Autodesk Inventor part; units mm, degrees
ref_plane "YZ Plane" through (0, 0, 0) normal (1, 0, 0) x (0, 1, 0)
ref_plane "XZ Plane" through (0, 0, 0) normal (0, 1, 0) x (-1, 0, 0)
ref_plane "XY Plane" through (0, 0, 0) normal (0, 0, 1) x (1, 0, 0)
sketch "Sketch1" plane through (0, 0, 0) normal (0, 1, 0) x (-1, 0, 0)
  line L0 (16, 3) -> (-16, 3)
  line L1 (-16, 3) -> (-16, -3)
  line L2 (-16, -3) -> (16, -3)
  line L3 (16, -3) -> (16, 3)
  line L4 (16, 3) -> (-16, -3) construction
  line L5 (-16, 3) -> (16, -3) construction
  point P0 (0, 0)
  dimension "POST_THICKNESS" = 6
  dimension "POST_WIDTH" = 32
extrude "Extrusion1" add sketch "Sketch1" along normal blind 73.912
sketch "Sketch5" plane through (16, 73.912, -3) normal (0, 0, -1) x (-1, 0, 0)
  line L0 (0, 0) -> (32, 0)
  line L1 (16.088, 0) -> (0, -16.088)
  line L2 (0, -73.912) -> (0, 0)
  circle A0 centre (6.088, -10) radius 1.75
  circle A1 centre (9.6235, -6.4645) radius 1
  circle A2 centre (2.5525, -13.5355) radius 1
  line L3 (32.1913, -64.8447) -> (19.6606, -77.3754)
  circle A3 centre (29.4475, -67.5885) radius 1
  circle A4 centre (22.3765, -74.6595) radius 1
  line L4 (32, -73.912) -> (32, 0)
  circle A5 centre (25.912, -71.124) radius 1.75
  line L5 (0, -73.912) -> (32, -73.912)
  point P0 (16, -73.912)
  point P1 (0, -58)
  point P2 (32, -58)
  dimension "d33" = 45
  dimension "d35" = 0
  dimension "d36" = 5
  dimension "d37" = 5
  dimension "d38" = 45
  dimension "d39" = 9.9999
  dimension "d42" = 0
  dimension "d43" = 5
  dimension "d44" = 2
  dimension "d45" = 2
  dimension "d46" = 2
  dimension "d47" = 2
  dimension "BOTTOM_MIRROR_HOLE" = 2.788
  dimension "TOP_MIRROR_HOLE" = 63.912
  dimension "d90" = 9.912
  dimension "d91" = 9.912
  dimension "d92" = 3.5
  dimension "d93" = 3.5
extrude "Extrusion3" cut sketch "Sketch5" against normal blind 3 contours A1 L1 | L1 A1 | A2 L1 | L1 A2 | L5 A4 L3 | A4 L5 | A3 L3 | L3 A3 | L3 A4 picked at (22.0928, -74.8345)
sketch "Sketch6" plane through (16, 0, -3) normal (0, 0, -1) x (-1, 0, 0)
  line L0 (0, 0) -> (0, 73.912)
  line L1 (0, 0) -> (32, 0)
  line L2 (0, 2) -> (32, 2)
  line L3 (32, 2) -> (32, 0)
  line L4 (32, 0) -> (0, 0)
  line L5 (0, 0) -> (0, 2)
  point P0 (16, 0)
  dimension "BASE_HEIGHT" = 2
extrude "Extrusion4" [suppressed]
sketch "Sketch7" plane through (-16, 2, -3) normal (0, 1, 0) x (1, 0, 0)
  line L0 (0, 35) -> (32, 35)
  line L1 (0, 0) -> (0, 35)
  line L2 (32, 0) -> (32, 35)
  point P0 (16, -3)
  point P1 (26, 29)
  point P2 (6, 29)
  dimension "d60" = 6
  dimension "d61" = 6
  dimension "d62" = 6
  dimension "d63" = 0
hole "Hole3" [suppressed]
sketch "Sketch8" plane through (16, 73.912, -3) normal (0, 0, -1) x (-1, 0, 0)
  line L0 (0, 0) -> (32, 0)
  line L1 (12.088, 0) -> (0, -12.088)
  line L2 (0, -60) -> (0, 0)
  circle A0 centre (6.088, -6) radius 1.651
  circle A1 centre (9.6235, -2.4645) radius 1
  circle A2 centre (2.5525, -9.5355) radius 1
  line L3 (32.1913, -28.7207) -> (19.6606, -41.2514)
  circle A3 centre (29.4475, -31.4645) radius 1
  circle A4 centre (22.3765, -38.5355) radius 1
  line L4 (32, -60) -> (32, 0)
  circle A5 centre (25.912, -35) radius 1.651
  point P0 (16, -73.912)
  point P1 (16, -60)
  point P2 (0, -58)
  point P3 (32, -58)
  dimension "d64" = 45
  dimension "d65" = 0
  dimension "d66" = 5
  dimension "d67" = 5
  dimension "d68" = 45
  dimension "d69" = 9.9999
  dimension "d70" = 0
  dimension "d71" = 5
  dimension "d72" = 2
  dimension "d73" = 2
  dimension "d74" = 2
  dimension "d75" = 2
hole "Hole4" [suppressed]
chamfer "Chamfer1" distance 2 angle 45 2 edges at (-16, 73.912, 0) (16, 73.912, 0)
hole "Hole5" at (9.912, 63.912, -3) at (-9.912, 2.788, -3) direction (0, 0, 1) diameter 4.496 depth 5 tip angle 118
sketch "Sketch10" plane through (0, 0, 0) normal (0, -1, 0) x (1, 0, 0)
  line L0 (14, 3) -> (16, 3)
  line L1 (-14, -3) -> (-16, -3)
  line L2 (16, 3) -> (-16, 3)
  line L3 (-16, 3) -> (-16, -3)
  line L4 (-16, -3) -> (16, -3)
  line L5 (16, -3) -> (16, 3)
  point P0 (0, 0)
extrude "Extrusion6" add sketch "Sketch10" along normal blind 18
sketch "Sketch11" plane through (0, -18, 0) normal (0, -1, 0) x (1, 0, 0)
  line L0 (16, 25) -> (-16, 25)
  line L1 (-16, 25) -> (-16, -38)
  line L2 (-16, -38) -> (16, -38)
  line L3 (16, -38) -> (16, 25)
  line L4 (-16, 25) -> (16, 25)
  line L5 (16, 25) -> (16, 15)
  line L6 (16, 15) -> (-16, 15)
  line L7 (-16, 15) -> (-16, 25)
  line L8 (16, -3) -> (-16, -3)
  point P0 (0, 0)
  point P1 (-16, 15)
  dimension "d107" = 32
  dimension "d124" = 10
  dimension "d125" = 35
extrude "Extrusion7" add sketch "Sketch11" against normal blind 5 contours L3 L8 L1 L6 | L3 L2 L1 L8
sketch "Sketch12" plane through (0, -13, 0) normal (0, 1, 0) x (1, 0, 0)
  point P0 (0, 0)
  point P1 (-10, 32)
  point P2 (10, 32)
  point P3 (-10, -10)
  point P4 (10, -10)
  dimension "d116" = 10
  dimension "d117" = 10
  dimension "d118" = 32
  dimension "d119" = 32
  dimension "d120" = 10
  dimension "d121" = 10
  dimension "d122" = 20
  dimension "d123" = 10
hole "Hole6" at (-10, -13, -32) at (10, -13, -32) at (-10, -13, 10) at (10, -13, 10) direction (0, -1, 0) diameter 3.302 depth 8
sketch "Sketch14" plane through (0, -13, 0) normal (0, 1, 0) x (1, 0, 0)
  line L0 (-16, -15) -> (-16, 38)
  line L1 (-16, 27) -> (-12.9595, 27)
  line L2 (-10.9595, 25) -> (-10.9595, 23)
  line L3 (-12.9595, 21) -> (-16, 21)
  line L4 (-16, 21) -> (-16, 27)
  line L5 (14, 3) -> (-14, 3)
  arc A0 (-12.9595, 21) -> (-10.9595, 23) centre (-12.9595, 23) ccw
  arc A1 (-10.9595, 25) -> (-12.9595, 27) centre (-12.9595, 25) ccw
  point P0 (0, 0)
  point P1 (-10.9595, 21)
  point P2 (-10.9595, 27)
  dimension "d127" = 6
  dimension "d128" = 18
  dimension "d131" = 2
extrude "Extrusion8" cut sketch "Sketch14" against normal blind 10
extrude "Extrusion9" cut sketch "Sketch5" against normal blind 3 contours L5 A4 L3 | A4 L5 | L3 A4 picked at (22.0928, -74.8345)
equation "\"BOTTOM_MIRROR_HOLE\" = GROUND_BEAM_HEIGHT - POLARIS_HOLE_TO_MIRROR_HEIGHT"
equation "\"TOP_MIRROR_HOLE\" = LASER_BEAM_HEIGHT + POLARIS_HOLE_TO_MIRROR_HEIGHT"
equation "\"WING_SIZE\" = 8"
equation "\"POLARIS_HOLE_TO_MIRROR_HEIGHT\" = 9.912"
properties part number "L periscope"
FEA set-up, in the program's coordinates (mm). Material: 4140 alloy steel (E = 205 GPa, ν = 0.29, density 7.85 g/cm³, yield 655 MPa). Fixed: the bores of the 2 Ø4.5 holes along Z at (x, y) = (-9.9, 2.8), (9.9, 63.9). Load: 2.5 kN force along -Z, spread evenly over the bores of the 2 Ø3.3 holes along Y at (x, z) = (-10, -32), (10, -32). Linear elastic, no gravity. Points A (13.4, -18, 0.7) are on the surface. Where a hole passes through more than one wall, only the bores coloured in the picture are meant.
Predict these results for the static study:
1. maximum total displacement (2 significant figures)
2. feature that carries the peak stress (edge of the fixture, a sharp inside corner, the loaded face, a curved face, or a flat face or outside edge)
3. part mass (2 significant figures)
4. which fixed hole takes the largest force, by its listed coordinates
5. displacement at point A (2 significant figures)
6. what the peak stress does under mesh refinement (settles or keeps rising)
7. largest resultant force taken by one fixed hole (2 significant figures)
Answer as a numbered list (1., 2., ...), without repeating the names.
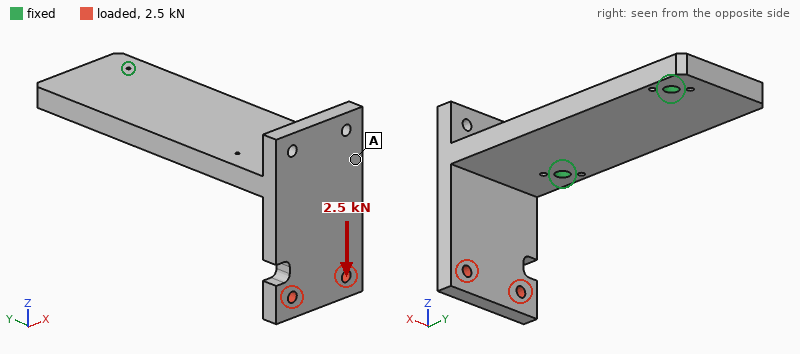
1. 0.27 mm
2. edge of the fixture
3. 190 g
4. (-9.9, 2.8)
5. 0.14 mm
6. keeps rising
7. 2.7 kN
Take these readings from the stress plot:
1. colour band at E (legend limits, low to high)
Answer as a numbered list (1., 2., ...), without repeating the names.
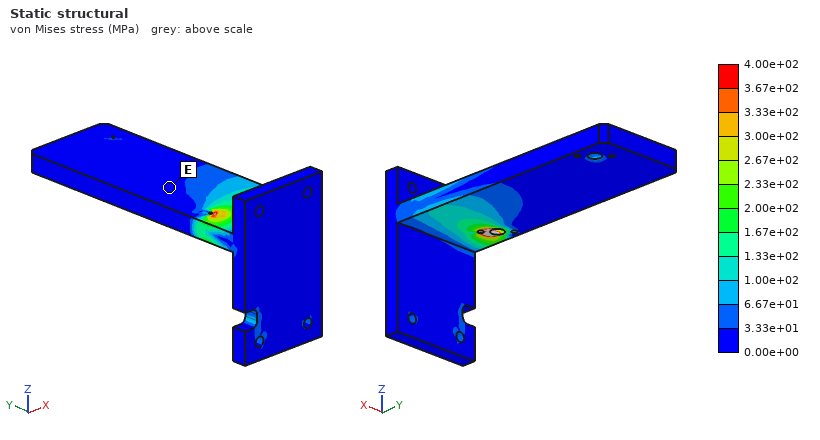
1. 0.00e+00 to 3.33e+01 MPa
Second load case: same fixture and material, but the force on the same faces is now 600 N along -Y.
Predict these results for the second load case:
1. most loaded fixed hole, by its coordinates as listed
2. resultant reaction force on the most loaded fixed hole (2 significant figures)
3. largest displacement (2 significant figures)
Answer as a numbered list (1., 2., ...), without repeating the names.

1. (-9.9, 2.8)
2. 510 N
3. 0.25 mm
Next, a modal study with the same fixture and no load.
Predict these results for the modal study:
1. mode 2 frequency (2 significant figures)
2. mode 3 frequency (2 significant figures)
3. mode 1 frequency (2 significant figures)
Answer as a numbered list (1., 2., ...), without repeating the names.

1. 2400 Hz
2. 5000 Hz
3. 1800 Hz
